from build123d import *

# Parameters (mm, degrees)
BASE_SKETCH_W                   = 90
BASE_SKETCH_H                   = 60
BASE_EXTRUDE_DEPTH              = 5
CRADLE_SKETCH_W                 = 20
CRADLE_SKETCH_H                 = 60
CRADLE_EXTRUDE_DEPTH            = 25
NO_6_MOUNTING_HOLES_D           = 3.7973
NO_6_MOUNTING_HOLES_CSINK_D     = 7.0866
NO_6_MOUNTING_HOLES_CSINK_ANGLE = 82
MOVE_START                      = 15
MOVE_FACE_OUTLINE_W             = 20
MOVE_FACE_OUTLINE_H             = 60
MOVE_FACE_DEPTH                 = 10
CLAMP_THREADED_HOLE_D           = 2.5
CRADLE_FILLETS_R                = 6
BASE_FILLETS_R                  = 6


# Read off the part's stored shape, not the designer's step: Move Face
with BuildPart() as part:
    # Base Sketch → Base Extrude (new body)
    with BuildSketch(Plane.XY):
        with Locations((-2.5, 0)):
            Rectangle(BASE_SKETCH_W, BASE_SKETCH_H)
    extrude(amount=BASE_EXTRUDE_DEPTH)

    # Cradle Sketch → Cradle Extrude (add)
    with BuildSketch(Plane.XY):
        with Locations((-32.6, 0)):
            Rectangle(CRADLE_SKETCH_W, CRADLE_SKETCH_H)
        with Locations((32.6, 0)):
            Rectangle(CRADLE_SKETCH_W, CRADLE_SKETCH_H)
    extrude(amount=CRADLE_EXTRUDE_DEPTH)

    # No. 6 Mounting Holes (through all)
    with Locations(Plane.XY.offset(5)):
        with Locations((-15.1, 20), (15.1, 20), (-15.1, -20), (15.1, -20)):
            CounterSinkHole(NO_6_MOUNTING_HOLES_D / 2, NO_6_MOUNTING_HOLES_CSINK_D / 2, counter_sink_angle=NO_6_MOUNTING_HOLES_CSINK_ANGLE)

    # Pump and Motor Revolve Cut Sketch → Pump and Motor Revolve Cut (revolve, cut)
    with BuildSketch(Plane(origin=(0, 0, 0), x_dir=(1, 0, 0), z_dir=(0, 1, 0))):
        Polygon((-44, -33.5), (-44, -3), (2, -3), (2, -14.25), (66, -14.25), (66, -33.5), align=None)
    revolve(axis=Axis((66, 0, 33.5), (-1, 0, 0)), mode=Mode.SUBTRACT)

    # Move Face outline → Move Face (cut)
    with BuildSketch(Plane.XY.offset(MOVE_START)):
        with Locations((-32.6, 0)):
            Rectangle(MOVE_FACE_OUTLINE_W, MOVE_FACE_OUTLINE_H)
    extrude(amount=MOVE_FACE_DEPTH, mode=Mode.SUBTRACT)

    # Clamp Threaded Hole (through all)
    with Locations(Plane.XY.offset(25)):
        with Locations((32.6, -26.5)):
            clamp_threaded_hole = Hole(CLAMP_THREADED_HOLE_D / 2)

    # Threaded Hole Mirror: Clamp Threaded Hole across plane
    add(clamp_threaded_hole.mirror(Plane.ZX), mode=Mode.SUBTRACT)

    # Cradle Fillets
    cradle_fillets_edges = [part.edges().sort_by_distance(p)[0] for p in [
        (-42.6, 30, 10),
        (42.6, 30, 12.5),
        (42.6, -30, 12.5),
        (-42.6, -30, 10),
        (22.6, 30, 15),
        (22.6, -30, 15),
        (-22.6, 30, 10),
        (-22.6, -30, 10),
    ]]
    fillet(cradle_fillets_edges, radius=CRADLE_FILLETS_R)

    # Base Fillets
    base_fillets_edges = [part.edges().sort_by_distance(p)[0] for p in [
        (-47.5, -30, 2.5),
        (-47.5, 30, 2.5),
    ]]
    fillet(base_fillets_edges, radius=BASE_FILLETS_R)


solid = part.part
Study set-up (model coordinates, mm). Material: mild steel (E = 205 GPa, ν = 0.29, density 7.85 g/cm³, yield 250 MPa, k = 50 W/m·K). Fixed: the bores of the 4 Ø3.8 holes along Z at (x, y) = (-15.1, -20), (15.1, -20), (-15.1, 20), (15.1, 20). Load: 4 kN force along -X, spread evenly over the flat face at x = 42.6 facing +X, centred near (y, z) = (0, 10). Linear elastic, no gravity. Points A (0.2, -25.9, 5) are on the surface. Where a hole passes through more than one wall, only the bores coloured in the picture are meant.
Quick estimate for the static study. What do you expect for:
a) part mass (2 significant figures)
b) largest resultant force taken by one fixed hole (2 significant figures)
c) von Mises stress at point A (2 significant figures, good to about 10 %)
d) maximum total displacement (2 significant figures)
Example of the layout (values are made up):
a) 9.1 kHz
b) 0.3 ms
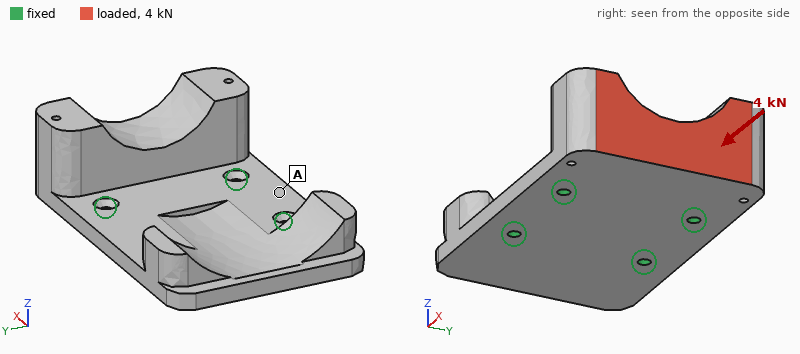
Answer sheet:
a) 370 g
b) 1.1 kN
c) 24 MPa
d) 0.11 mm
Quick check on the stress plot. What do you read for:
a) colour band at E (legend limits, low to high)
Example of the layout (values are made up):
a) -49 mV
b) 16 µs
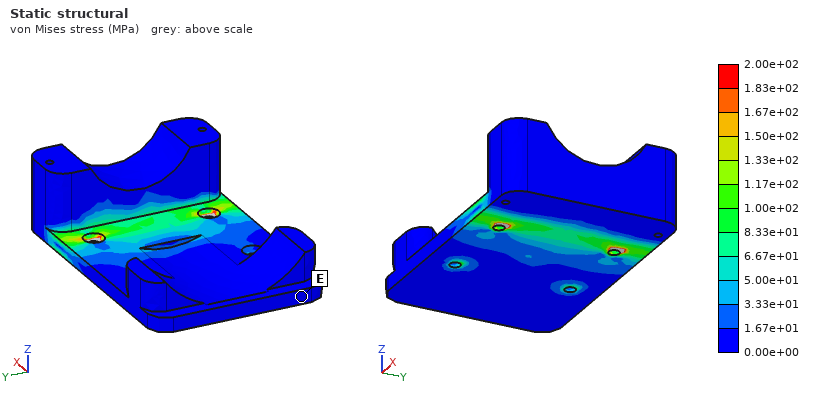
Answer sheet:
a) 0.00e+00 to 1.67e+01 MPa
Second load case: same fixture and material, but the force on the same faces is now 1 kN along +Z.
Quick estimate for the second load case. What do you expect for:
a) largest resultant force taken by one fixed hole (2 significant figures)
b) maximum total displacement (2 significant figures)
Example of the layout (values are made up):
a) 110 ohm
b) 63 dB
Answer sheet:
a) 860 N
b) 86 µm
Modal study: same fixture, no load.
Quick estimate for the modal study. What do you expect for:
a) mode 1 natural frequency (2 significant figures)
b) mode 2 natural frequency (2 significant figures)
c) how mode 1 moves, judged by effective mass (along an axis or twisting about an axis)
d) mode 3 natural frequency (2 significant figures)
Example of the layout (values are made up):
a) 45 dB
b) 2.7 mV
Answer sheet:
a) 1900 Hz
b) 2700 Hz
c) along Z
d) 4400 Hz
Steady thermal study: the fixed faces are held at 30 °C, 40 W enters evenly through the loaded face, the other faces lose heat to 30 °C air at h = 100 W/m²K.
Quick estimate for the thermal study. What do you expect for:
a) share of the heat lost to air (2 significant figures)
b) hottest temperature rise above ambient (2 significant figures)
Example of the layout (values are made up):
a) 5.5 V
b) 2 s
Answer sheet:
a) 46 %
b) 40 K
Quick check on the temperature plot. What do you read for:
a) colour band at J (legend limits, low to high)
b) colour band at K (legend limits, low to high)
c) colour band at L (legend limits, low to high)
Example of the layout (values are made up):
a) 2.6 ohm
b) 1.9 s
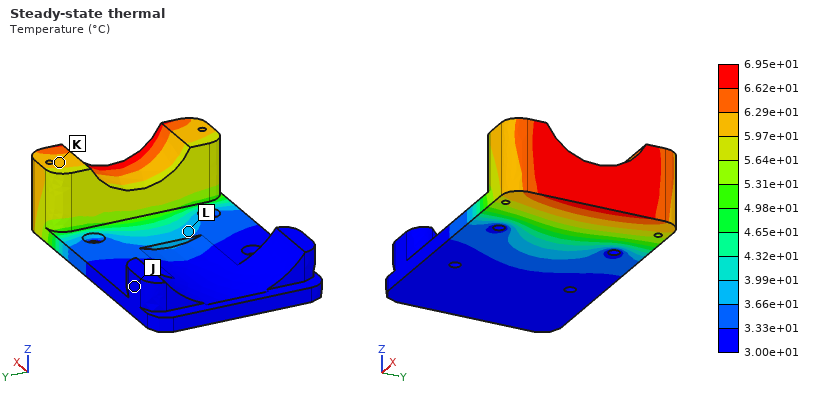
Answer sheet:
a) 3.00e+01 to 3.33e+01 °C
b) 5.97e+01 to 6.29e+01 °C
c) 3.66e+01 to 3.99e+01 °C
